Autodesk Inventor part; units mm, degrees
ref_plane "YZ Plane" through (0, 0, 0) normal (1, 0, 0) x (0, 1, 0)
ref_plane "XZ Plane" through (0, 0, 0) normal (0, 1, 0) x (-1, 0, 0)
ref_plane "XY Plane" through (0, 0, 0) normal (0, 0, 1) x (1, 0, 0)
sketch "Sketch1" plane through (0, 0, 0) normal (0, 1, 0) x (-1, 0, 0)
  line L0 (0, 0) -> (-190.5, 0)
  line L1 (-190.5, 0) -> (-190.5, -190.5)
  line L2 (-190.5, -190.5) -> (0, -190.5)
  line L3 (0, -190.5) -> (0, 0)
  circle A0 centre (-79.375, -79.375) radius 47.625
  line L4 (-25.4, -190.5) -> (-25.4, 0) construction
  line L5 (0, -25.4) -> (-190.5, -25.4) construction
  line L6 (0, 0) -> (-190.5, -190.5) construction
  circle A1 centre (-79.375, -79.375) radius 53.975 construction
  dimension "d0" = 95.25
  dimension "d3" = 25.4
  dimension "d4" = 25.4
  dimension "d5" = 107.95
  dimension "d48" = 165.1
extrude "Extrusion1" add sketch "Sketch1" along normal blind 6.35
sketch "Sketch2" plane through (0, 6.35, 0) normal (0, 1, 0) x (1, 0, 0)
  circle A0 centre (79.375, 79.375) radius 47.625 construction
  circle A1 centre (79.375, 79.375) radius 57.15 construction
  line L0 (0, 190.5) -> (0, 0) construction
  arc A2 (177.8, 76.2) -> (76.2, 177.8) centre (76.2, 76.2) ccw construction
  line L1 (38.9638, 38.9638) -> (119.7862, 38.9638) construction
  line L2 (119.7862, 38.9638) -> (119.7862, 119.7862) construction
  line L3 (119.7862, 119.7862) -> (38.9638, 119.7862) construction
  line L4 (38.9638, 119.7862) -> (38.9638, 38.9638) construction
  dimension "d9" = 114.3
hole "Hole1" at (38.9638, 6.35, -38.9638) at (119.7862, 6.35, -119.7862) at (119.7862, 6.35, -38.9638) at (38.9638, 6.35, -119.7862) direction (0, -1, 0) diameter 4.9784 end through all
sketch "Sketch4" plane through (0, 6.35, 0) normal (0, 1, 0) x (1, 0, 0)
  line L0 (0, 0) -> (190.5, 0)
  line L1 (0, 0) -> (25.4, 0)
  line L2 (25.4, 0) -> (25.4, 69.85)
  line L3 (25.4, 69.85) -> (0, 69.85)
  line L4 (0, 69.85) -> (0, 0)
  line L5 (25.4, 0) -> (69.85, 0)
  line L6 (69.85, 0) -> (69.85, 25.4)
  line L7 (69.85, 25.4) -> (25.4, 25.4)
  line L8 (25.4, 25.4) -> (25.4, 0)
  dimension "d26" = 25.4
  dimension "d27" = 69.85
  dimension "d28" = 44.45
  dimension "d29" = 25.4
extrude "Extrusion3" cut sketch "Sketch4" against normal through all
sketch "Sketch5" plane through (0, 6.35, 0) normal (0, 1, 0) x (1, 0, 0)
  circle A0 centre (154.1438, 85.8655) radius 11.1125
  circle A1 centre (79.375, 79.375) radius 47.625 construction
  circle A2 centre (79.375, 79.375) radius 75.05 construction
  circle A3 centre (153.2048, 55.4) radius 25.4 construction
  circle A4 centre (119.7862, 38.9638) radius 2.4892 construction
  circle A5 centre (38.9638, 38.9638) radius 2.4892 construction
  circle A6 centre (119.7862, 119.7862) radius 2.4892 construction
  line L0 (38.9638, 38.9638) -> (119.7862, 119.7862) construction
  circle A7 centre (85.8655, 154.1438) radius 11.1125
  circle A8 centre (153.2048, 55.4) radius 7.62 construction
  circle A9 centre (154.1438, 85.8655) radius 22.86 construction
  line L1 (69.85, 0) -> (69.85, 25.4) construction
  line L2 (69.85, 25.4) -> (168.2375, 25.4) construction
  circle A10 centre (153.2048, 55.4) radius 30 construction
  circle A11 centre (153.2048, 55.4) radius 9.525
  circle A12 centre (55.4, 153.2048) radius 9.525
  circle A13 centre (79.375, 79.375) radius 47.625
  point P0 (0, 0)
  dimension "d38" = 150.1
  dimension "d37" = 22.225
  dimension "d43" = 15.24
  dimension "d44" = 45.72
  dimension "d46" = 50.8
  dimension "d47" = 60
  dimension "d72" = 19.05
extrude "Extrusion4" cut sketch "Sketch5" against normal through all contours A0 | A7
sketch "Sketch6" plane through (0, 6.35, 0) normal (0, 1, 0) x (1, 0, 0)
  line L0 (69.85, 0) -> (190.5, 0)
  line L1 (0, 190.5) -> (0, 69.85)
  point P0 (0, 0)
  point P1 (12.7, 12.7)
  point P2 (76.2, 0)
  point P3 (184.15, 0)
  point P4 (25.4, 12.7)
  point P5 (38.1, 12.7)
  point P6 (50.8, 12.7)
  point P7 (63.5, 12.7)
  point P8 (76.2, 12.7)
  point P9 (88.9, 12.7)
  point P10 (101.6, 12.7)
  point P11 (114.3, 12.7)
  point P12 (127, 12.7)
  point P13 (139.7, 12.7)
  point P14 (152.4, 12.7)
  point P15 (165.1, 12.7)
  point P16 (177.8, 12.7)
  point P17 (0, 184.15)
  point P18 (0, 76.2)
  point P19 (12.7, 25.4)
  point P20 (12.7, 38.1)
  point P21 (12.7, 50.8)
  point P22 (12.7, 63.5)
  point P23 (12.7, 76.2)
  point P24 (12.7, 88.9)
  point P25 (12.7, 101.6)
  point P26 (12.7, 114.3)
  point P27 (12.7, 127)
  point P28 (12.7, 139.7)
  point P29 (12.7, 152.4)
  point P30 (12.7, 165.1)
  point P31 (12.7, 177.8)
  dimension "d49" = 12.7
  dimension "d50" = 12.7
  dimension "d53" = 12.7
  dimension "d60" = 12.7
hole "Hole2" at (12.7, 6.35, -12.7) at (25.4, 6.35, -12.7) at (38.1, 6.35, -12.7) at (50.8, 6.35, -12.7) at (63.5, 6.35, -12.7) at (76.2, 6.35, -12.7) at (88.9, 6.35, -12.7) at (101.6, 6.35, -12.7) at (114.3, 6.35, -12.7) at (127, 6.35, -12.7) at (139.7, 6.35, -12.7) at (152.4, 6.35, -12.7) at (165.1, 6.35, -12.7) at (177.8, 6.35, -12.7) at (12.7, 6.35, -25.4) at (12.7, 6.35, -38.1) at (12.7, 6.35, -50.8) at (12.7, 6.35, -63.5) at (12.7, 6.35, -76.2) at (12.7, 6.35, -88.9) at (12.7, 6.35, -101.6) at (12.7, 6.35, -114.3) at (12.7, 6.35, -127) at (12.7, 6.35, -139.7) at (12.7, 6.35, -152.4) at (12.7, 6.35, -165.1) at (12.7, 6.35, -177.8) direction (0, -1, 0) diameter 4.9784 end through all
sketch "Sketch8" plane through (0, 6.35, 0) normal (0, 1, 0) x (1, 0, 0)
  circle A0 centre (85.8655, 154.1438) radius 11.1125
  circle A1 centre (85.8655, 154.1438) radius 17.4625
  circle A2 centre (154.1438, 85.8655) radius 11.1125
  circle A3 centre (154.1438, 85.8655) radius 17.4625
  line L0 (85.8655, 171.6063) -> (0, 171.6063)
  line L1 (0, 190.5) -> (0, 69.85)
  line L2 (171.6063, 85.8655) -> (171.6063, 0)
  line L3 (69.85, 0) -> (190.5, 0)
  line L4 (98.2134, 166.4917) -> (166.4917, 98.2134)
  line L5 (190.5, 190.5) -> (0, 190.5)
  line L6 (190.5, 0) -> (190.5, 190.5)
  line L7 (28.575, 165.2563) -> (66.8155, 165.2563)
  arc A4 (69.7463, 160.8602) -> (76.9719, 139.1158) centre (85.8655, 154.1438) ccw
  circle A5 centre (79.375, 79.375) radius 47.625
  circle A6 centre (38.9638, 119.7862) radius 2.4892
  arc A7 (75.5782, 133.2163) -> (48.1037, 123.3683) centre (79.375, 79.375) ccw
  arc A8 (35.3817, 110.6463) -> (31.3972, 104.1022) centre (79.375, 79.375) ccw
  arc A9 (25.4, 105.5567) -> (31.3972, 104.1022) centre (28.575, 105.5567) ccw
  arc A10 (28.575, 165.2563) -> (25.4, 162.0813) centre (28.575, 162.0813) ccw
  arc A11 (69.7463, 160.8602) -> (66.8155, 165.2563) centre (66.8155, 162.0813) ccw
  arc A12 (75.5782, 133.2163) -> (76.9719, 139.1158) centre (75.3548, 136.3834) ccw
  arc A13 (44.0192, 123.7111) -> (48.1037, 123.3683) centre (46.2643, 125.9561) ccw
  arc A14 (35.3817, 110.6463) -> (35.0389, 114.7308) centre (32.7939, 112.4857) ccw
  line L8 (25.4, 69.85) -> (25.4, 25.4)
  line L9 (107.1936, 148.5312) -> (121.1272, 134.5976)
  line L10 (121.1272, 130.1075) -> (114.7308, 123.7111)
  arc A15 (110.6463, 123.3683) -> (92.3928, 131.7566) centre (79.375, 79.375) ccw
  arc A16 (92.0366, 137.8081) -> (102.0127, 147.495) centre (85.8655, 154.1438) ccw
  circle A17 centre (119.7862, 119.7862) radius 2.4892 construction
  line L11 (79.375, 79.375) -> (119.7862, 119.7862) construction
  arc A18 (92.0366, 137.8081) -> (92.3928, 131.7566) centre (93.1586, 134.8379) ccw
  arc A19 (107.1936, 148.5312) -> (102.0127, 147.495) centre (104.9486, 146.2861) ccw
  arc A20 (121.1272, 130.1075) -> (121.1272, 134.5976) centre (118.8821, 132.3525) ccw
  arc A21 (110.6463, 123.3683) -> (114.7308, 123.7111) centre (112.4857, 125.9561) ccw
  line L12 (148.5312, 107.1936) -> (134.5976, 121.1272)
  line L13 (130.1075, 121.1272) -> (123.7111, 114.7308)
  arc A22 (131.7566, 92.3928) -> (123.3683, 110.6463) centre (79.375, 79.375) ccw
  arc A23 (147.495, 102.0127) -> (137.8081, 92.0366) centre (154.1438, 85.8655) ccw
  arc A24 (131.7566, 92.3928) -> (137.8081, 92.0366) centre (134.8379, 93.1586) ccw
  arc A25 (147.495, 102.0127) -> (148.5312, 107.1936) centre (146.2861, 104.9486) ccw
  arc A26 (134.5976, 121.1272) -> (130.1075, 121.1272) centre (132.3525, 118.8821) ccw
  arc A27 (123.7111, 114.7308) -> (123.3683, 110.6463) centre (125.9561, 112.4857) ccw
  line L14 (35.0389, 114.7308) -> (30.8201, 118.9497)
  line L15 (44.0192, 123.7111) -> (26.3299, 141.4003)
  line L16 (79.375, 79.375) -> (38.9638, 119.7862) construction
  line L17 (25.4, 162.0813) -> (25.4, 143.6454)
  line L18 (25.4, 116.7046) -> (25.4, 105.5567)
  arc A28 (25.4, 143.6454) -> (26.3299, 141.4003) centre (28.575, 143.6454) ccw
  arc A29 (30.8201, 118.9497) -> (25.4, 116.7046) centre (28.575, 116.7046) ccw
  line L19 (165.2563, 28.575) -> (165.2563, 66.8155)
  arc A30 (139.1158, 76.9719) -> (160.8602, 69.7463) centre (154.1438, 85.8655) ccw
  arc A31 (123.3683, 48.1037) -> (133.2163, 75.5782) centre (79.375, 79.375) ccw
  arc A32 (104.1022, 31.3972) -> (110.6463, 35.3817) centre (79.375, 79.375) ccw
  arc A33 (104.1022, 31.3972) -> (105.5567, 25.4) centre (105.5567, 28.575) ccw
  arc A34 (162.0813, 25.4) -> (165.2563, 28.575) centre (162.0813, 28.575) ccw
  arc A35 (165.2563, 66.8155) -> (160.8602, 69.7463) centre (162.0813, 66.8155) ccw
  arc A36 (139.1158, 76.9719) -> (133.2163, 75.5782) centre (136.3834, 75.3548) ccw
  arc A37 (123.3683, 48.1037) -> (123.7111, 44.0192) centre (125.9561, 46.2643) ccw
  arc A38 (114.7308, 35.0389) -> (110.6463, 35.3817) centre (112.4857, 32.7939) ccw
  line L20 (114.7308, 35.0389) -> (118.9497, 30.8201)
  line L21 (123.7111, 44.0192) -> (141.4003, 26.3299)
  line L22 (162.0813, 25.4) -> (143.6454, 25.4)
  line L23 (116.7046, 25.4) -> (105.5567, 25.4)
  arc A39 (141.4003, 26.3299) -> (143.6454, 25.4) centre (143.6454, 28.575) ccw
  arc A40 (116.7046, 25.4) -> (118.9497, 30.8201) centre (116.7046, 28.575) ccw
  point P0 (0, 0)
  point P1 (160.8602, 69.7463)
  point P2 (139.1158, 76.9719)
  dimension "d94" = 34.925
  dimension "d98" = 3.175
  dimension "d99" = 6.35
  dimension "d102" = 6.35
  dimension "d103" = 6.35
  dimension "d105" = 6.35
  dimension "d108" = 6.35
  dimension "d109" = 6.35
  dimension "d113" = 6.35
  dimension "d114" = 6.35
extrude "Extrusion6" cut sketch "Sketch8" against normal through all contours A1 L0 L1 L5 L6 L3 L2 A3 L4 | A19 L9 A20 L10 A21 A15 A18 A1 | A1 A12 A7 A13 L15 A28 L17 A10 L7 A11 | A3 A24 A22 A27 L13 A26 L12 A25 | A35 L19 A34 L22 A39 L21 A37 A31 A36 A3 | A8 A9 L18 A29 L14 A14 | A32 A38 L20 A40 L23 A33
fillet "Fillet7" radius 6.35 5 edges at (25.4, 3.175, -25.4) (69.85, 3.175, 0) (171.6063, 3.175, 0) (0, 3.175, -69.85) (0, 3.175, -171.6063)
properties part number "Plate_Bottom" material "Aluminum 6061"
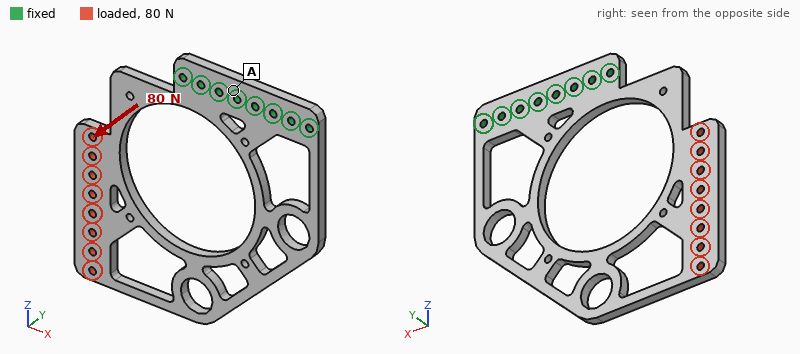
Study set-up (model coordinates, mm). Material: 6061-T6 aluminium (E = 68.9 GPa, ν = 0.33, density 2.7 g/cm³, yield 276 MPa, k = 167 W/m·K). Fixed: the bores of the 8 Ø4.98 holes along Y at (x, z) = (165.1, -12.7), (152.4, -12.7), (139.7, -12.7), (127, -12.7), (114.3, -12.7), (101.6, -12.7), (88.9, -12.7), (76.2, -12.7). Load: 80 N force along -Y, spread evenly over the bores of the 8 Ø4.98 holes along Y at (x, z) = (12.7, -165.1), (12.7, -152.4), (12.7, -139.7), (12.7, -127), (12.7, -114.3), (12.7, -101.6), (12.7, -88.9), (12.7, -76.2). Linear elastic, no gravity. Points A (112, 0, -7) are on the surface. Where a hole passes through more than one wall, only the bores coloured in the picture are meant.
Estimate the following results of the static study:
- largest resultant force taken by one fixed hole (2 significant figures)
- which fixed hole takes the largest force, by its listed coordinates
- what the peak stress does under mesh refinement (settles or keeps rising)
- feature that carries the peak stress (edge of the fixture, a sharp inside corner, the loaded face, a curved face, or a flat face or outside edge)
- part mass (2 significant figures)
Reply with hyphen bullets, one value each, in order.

- 200 N
- (76.2, -12.7)
- keeps rising
- a sharp inside corner
- 180 g
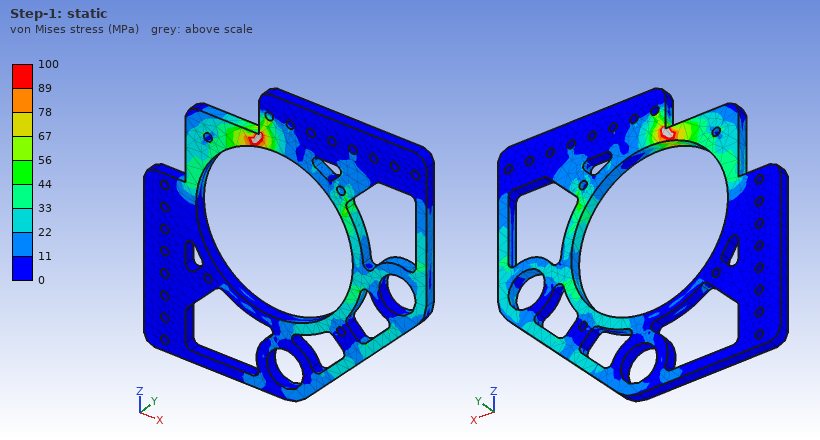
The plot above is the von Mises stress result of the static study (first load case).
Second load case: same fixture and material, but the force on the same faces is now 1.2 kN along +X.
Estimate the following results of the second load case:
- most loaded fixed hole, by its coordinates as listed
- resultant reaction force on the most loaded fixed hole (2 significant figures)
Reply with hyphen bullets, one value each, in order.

- (165.1, -12.7)
- 2.0 kN
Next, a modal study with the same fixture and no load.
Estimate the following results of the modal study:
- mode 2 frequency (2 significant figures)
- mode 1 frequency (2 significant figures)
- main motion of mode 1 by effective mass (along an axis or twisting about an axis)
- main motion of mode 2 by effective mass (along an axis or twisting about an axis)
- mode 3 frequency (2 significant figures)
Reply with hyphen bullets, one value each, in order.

- 330 Hz
- 120 Hz
- along Y
- twisting about Z
- 730 Hz
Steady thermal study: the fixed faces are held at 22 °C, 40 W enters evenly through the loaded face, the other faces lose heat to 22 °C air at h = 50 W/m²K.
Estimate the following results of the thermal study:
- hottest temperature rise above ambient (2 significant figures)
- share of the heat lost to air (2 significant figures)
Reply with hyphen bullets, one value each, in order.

- 58 K
- 85 %
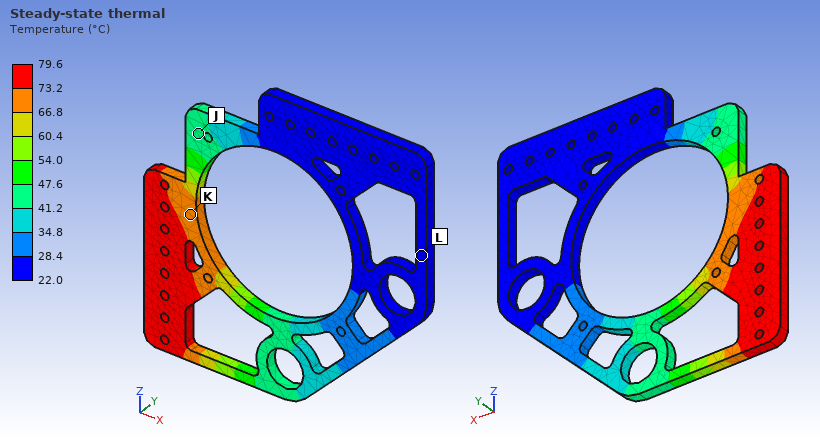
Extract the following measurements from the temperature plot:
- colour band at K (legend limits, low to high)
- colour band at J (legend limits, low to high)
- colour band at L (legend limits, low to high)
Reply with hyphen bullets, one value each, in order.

- 66.8 to 73.2 °C
- 41.2 to 47.6 °C
- 22.0 to 28.4 °C
